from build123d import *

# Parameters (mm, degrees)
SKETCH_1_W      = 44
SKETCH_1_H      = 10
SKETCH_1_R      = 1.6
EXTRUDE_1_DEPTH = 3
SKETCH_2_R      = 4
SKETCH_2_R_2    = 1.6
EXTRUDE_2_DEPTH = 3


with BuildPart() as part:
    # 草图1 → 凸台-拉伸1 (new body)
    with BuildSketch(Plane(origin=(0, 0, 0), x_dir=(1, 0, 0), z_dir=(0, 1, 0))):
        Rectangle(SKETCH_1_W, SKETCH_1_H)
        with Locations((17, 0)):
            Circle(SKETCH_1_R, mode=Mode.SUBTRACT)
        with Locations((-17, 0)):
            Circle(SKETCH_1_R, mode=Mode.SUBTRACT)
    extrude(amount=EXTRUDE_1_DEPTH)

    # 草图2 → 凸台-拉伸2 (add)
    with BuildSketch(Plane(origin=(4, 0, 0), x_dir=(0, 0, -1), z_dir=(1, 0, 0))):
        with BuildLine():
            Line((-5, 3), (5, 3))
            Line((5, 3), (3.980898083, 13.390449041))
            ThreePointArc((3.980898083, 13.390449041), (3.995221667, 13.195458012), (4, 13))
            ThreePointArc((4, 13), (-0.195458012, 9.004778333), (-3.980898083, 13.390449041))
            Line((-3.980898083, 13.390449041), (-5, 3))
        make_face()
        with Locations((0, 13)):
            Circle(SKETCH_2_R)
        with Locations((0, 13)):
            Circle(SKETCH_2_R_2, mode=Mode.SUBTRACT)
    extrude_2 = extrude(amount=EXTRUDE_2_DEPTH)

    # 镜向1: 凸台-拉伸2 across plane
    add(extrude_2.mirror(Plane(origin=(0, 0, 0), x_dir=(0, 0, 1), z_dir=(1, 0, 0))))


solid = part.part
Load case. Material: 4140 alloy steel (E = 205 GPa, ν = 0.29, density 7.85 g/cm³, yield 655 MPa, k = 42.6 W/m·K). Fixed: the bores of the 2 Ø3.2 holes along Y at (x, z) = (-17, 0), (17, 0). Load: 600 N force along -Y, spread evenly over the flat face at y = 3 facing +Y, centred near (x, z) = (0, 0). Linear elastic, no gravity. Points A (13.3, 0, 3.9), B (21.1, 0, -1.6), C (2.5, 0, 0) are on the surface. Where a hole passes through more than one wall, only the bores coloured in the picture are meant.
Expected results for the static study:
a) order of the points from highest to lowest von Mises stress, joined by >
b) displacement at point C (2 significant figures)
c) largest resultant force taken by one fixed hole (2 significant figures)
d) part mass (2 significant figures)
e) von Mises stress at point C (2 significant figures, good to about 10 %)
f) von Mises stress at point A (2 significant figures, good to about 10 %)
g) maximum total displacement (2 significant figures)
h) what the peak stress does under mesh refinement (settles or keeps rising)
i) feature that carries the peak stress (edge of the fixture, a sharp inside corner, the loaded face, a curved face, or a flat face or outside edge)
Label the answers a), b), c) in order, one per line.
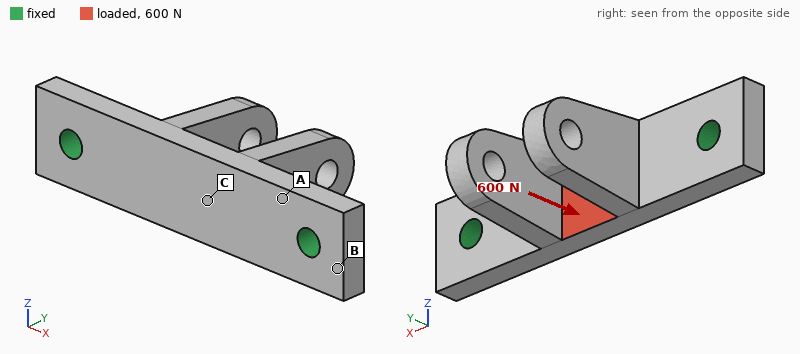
a) C > A > B
b) 22 µm
c) 300 N
d) 15 g
e) 100 MPa
f) 81 MPa
g) 35 µm
h) keeps rising
i) edge of the fixture
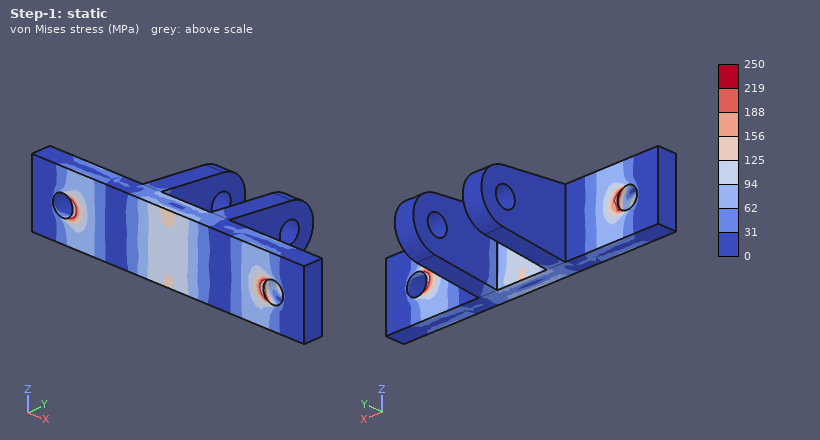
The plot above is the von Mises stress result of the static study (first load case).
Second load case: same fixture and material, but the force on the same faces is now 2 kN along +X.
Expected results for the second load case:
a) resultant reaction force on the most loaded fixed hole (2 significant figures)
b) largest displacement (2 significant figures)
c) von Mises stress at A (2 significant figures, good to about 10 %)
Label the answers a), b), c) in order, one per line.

a) 1.0 kN
b) 4.1 µm
c) 35 MPa
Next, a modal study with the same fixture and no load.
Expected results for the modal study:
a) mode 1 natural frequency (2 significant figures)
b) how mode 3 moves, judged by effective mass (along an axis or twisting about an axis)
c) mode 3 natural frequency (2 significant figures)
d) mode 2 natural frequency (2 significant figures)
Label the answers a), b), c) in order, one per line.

a) 8200 Hz
b) along X
c) 12 kHz
d) 8400 Hz
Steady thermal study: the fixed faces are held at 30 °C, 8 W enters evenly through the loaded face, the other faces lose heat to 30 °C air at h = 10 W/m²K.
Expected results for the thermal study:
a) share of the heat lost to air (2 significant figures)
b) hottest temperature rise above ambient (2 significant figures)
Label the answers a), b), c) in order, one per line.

a) 4.8 %
b) 45 K
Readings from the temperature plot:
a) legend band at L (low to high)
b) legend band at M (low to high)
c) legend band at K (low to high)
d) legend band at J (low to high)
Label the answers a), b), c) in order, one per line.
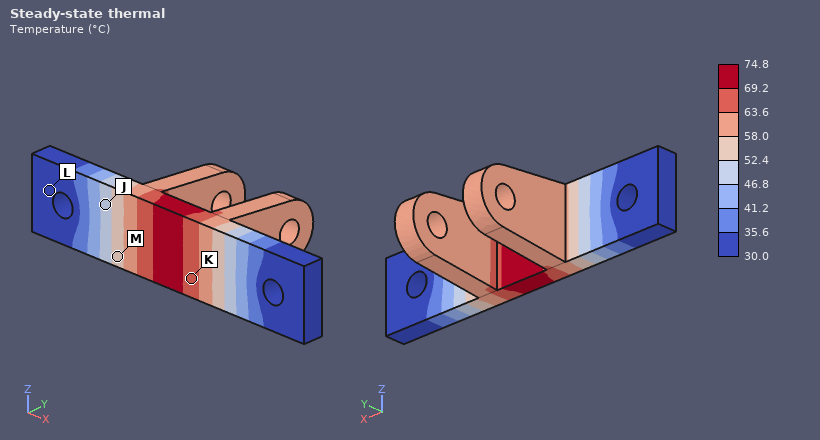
a) 30.0 to 35.6 °C
b) 52.4 to 58.0 °C
c) 63.6 to 69.2 °C
d) 46.8 to 52.4 °C
